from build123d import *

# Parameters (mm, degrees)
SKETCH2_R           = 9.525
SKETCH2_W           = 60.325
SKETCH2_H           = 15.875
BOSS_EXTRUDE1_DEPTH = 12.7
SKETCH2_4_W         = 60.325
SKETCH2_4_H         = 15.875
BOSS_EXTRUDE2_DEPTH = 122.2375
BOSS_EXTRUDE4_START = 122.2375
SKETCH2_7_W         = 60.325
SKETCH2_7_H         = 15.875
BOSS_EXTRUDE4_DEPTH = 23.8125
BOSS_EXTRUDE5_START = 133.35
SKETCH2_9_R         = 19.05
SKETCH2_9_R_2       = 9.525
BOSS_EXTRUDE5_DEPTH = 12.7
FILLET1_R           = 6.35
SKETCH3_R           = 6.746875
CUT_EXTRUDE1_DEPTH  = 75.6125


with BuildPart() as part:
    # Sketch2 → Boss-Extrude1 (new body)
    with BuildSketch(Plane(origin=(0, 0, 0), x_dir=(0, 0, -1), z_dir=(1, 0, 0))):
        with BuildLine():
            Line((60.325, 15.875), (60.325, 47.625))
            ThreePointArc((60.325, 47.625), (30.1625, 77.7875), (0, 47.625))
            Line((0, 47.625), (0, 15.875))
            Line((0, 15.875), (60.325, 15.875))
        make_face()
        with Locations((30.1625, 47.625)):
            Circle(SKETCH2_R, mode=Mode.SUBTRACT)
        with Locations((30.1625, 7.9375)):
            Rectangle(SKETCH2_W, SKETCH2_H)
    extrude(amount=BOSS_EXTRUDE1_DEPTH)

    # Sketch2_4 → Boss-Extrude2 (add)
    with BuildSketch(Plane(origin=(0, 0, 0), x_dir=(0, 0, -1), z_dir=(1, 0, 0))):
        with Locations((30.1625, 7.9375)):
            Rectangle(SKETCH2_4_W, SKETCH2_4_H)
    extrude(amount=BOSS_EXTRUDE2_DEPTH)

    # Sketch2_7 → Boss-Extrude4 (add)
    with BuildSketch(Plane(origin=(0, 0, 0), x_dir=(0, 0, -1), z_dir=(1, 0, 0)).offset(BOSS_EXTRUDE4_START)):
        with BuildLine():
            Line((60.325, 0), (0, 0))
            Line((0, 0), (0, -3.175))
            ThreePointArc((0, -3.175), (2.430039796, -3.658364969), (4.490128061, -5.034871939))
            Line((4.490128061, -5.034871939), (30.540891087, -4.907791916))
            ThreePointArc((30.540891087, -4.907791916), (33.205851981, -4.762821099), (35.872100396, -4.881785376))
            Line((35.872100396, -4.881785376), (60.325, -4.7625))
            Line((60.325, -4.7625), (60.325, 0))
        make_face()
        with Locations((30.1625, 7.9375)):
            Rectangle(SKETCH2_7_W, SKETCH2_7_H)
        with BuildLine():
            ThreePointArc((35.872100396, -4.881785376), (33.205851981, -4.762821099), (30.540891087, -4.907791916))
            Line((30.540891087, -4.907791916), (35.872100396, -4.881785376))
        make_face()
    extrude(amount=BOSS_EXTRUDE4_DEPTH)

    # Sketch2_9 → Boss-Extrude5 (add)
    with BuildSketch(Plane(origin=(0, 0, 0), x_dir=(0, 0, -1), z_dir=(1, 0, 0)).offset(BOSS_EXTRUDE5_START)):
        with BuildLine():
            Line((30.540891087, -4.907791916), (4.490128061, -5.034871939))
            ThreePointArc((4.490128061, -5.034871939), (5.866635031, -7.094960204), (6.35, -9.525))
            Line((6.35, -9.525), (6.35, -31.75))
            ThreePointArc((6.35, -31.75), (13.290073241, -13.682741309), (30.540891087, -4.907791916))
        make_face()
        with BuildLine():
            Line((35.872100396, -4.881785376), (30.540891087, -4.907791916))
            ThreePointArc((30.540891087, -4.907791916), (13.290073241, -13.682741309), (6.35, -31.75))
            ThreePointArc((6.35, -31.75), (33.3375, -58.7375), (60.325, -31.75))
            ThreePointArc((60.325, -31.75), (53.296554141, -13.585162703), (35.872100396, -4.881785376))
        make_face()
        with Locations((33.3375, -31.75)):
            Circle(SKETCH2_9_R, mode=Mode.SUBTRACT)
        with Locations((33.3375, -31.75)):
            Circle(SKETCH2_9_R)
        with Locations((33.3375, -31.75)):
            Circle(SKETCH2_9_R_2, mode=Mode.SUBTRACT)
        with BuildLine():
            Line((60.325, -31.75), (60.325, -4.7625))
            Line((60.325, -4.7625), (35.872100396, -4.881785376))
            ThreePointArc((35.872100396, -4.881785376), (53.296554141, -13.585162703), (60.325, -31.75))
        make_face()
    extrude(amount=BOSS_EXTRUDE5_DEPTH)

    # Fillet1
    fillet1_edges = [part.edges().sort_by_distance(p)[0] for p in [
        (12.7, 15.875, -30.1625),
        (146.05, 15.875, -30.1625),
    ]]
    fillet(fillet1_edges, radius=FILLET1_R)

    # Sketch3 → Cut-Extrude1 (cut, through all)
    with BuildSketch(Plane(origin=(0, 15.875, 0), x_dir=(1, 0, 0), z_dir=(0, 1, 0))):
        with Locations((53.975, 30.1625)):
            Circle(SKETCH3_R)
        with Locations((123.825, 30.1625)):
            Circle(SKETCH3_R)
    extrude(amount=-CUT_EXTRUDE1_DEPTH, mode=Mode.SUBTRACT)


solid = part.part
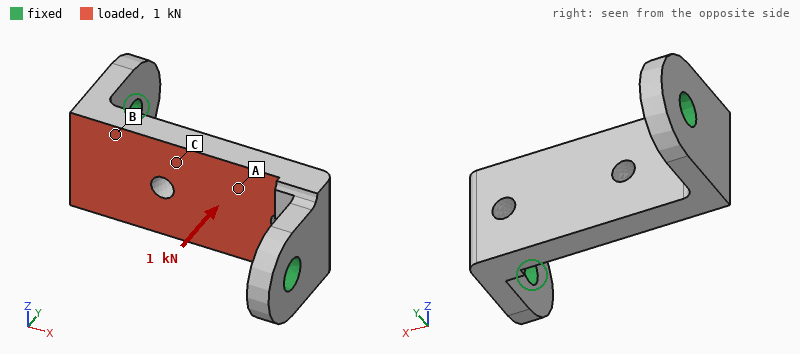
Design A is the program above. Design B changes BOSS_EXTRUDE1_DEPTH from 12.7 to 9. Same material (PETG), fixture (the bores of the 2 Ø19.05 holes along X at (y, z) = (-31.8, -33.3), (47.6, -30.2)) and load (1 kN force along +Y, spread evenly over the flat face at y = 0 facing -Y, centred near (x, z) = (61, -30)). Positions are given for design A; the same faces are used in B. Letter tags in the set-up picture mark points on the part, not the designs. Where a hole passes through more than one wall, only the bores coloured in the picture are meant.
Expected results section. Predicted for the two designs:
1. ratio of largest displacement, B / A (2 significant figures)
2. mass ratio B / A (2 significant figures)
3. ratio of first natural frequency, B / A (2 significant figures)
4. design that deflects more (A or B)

1.2
0.95
0.90
B
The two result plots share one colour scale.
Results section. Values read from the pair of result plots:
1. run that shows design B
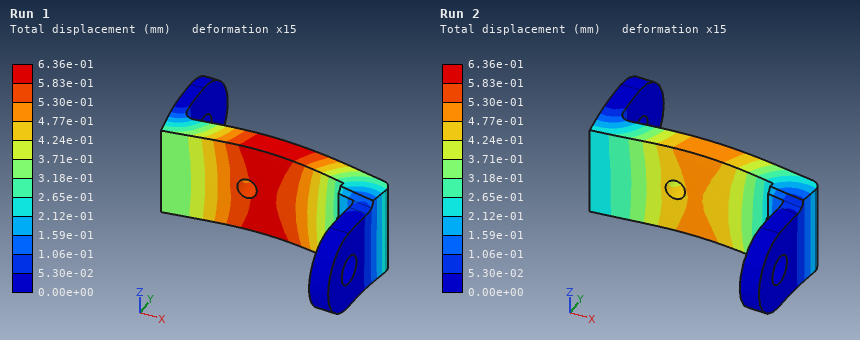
Run 1
